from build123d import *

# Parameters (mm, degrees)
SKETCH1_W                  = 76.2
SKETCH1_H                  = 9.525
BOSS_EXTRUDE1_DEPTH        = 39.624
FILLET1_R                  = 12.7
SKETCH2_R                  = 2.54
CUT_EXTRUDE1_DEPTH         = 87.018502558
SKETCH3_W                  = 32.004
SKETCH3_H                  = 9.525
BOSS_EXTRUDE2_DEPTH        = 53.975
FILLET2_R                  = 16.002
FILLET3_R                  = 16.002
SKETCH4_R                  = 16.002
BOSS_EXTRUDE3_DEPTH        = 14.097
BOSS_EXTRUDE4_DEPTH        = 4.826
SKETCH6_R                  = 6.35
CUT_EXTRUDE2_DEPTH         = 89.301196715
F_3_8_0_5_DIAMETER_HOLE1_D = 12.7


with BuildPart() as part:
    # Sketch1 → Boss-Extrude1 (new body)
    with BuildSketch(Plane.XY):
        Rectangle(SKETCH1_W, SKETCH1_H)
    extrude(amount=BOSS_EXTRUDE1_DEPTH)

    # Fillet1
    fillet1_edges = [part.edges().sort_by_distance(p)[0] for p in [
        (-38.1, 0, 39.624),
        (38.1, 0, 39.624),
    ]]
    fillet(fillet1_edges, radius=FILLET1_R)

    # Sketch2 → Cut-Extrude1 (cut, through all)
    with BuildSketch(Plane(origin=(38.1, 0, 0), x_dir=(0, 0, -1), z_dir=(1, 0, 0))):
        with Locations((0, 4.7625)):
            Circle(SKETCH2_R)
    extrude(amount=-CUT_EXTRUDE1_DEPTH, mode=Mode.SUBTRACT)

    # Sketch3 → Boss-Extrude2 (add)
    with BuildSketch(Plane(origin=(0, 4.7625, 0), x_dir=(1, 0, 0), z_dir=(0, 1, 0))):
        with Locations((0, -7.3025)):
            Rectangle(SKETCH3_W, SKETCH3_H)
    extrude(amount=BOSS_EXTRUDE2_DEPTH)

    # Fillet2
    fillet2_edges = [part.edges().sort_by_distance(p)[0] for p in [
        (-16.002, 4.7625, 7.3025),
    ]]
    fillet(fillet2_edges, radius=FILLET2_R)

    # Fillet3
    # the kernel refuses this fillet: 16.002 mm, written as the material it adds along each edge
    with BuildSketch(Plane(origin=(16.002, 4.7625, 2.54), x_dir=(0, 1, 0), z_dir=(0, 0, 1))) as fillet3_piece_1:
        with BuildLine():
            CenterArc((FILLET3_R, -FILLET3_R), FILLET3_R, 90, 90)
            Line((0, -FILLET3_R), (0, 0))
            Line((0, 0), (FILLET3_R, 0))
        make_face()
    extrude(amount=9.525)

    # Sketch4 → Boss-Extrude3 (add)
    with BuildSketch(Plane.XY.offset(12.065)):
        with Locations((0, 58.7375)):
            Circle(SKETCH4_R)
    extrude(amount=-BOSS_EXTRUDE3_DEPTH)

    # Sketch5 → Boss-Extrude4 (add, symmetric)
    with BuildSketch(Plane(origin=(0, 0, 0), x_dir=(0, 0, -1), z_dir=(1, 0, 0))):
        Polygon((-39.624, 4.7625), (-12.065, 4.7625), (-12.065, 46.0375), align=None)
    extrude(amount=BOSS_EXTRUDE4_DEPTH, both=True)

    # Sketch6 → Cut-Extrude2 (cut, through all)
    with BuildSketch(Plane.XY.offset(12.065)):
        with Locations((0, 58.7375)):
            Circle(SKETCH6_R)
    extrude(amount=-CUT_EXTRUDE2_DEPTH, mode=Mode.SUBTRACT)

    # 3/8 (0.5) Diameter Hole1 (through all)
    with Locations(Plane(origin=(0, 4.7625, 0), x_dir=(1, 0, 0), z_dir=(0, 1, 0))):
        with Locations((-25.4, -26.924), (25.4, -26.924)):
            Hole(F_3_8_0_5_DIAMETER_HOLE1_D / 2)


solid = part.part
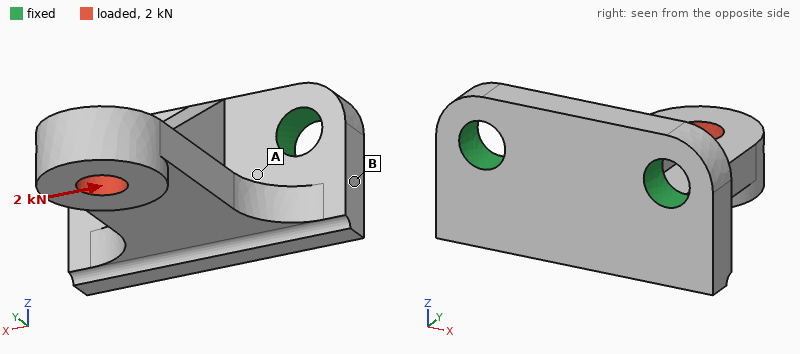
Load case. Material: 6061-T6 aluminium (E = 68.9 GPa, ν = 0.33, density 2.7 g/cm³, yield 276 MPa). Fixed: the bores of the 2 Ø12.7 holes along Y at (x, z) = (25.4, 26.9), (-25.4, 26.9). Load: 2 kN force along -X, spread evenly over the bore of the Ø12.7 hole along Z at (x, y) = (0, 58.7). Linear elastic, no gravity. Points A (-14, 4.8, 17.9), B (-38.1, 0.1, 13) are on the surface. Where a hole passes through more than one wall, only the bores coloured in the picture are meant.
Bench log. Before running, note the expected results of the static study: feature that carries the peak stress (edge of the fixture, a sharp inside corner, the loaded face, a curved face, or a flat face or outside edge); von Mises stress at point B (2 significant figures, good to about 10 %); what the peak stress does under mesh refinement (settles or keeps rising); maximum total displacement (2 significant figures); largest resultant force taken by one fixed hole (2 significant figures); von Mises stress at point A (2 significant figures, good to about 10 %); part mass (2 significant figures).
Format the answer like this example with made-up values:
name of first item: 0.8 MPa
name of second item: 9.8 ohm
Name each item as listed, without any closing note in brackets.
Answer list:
feature that carries the peak stress: edge of the fixture
von Mises stress at point B: 9.8 MPa
what the peak stress does under mesh refinement: keeps rising
maximum total displacement: 0.15 mm
largest resultant force taken by one fixed hole: 2.9 kN
von Mises stress at point A: 22 MPa
part mass: 150 g
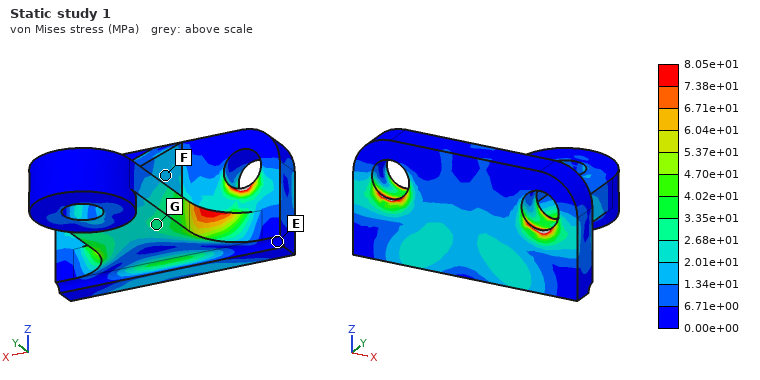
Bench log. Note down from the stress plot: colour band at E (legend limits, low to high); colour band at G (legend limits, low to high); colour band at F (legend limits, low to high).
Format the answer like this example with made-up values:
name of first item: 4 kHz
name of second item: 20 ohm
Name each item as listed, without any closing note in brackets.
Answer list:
colour band at E: 0.00e+00 to 6.71e+00 MPa
colour band at G: 2.68e+01 to 3.35e+01 MPa
colour band at F: 1.34e+01 to 2.01e+01 MPa
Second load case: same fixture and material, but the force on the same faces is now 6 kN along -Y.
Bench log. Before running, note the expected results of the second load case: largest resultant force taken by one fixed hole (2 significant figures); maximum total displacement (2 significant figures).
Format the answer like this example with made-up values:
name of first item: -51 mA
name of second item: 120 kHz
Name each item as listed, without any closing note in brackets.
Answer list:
largest resultant force taken by one fixed hole: 3.1 kN
maximum total displacement: 0.25 mm
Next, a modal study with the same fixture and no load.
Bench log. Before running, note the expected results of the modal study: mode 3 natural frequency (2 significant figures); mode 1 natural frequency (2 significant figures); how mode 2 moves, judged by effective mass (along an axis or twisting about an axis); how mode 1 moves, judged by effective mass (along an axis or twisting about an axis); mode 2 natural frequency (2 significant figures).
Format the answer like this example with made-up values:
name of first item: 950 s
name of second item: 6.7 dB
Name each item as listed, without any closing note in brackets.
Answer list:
mode 3 natural frequency: 7300 Hz
mode 1 natural frequency: 2300 Hz
how mode 2 moves, judged by effective mass: along X
how mode 1 moves, judged by effective mass: along Z
mode 2 natural frequency: 3700 Hz
